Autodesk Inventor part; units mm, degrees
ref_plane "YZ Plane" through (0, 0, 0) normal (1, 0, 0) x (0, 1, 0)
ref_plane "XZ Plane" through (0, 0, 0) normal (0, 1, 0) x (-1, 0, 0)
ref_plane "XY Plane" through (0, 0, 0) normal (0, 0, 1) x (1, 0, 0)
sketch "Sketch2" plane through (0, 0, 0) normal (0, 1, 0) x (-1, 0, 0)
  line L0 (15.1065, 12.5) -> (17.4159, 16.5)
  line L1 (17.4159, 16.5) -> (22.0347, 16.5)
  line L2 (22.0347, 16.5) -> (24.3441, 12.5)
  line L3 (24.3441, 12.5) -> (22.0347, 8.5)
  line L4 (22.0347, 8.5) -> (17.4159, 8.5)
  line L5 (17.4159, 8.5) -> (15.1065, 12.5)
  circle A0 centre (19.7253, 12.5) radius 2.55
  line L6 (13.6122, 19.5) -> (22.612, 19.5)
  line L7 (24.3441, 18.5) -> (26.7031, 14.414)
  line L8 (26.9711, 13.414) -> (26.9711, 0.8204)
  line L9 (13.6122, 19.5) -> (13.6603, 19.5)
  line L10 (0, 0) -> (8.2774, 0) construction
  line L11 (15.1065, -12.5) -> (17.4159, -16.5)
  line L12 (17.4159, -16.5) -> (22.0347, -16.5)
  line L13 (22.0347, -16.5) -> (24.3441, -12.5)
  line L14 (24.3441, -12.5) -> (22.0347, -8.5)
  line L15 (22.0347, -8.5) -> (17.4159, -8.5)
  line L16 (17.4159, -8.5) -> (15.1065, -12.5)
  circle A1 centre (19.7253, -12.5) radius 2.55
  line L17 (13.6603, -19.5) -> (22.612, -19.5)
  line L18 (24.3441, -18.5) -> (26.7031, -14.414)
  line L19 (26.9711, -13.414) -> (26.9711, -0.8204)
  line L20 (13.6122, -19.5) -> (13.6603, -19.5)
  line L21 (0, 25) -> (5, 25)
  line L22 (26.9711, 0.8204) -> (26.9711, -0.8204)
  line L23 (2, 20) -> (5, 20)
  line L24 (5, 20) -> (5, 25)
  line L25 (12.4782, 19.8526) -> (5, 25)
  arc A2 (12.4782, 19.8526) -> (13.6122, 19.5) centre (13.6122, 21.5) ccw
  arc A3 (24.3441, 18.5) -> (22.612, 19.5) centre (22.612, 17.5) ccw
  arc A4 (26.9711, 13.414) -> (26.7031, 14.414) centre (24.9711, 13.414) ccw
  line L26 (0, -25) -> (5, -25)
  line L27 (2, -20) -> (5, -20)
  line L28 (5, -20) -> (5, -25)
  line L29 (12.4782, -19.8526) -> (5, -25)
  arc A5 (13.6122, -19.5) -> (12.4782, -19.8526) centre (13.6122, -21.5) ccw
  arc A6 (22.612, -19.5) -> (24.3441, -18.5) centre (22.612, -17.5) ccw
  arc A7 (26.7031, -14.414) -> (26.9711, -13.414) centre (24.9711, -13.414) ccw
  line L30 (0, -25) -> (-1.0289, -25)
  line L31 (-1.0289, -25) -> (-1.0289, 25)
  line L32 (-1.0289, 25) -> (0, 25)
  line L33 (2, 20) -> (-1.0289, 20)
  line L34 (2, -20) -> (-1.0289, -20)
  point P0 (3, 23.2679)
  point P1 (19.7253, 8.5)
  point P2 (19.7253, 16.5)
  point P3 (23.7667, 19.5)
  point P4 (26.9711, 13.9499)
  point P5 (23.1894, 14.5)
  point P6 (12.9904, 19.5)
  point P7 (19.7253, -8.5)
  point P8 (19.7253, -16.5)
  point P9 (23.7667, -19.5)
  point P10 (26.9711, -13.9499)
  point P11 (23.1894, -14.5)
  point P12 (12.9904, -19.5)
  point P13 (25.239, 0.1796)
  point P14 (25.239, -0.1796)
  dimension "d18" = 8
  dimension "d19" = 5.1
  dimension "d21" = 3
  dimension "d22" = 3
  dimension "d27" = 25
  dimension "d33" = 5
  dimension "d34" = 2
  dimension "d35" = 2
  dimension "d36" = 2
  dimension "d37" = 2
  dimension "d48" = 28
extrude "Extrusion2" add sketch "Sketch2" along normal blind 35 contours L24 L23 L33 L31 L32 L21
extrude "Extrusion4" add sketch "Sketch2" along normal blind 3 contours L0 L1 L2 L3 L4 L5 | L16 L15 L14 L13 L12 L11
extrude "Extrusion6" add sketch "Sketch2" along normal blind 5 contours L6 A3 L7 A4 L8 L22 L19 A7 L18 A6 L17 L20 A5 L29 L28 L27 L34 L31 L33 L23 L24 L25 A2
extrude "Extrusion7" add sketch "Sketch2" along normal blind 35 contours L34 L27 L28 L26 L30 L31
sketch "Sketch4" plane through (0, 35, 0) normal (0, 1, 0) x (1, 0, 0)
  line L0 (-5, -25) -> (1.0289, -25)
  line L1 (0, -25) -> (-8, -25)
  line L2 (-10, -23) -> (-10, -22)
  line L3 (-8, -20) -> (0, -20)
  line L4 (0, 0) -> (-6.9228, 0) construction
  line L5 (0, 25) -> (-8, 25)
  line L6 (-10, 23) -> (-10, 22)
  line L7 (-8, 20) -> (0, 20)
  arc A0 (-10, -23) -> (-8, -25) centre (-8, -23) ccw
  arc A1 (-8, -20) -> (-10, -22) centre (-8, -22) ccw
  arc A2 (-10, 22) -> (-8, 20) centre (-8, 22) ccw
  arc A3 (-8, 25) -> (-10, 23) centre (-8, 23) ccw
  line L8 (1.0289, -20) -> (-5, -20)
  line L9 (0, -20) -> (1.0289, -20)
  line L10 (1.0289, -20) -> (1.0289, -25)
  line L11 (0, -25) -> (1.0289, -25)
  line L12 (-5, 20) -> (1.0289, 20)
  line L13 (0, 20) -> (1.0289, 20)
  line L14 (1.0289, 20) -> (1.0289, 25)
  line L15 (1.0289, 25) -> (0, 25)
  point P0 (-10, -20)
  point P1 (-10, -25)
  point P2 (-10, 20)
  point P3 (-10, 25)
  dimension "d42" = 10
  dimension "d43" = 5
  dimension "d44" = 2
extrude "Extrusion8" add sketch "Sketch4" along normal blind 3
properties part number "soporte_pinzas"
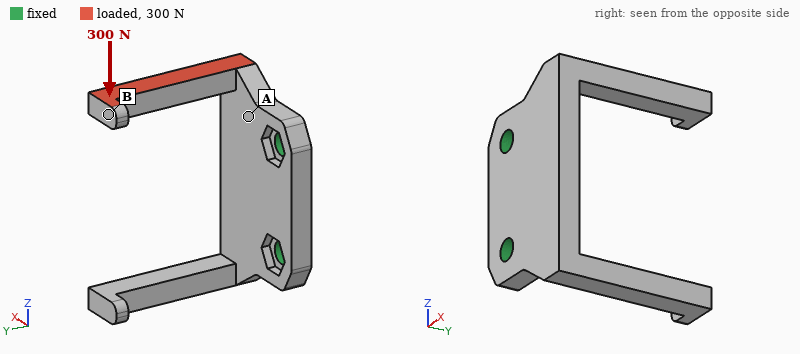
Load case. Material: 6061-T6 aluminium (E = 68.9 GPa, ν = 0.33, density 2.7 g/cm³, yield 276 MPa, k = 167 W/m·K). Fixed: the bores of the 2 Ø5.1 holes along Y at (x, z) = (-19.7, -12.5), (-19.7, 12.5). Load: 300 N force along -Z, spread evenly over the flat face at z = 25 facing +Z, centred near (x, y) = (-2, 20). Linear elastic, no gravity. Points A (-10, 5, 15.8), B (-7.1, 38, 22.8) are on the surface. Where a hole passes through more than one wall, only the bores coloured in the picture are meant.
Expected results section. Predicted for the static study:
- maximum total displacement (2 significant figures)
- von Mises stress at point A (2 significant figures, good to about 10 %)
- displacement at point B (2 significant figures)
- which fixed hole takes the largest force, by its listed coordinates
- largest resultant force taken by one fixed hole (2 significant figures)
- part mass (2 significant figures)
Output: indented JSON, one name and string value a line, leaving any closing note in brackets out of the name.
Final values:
{
  "maximum total displacement": "0.66 mm",
  "von Mises stress at point A": "83 MPa",
  "displacement at point B": "0.65 mm",
  "which fixed hole takes the largest force, by its listed coordinates": "(-19.7, -12.5)",
  "largest resultant force taken by one fixed hole": "380 N",
  "part mass": "21 g"
}
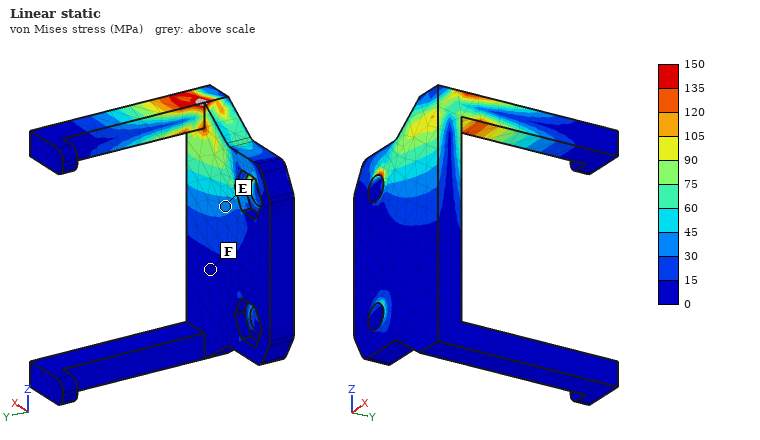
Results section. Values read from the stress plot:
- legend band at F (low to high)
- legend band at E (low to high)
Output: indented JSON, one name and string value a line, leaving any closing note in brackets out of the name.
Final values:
{
  "legend band at F": "0 to 15 MPa",
  "legend band at E": "30 to 45 MPa"
}
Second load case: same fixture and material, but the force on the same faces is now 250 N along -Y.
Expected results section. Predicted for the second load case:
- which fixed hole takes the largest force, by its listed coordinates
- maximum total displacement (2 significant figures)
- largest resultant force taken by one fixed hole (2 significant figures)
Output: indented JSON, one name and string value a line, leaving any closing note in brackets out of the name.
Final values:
{
  "which fixed hole takes the largest force, by its listed coordinates": "(-19.7, 12.5)",
  "maximum total displacement": "0.26 mm",
  "largest resultant force taken by one fixed hole": "340 N"
}
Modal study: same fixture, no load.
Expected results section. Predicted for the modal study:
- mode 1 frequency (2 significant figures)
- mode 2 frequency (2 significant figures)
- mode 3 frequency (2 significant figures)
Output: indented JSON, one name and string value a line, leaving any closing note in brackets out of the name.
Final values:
{
  "mode 1 frequency": "2100 Hz",
  "mode 2 frequency": "2100 Hz",
  "mode 3 frequency": "2200 Hz"
}
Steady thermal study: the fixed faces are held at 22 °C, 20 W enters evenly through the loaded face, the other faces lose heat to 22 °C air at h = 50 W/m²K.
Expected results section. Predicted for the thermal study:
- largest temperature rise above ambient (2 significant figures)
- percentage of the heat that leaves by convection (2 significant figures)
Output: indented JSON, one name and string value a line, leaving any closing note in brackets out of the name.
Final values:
{
  "largest temperature rise above ambient": "84 K",
  "percentage of the heat that leaves by convection": "15 %"
}
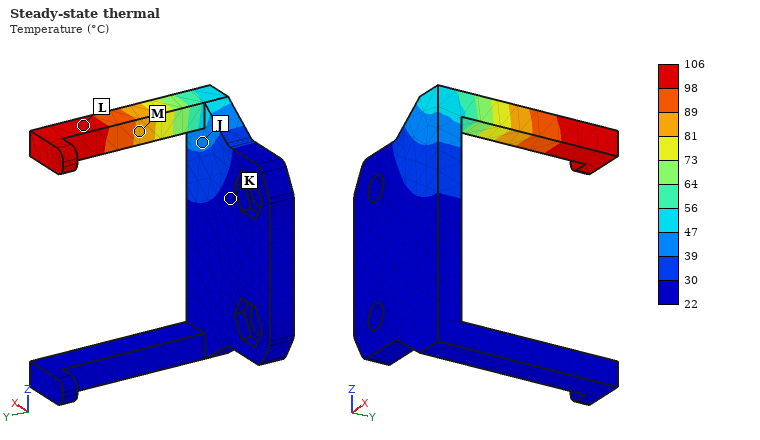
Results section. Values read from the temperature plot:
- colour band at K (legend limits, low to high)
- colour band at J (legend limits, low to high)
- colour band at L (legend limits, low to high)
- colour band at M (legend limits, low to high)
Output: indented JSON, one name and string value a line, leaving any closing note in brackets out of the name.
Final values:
{
  "colour band at K": "22 to 30 °C",
  "colour band at J": "39 to 47 °C",
  "colour band at L": "98 to 106 °C",
  "colour band at M": "81 to 89 °C"
}
